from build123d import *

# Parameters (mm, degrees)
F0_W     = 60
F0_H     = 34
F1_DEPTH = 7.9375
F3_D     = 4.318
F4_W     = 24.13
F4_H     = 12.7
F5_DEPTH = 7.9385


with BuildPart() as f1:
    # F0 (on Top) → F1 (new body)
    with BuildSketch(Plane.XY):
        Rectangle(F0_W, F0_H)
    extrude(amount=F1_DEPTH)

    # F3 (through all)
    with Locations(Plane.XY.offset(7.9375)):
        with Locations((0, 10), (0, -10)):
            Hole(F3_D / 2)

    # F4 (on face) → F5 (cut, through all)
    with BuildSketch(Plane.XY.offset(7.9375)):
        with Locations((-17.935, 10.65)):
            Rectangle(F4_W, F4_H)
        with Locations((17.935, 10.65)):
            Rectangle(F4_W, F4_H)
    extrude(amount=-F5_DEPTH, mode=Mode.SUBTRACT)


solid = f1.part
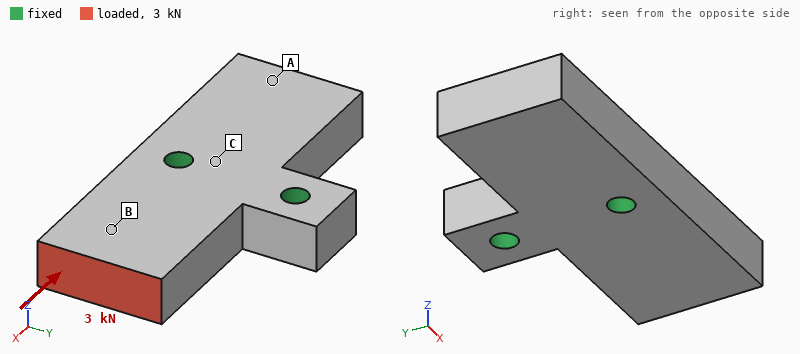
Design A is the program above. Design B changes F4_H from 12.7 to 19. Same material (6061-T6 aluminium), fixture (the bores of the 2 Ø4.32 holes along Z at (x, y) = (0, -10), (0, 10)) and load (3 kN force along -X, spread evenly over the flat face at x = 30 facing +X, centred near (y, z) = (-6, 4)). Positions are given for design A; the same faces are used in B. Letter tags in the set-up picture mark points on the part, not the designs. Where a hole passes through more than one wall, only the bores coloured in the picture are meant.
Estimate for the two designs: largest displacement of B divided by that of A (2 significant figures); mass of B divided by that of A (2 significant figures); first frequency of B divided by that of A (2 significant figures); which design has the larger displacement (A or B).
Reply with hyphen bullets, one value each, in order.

- 1.1
- 0.89
- 1.0
- B
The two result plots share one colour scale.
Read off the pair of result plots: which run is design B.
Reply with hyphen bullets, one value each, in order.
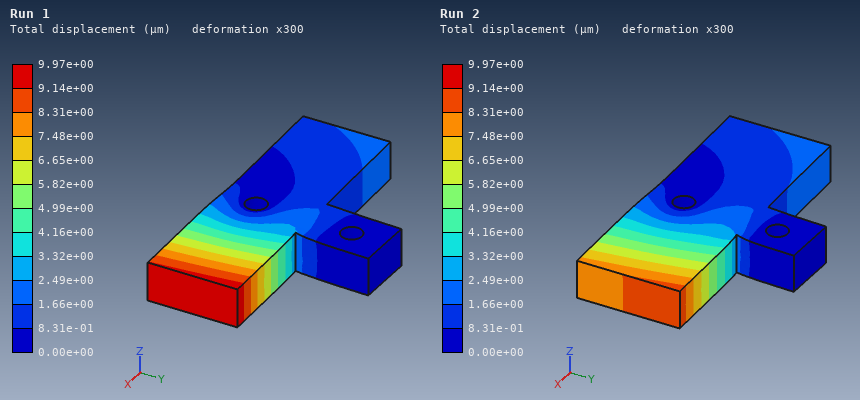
- Run 1
